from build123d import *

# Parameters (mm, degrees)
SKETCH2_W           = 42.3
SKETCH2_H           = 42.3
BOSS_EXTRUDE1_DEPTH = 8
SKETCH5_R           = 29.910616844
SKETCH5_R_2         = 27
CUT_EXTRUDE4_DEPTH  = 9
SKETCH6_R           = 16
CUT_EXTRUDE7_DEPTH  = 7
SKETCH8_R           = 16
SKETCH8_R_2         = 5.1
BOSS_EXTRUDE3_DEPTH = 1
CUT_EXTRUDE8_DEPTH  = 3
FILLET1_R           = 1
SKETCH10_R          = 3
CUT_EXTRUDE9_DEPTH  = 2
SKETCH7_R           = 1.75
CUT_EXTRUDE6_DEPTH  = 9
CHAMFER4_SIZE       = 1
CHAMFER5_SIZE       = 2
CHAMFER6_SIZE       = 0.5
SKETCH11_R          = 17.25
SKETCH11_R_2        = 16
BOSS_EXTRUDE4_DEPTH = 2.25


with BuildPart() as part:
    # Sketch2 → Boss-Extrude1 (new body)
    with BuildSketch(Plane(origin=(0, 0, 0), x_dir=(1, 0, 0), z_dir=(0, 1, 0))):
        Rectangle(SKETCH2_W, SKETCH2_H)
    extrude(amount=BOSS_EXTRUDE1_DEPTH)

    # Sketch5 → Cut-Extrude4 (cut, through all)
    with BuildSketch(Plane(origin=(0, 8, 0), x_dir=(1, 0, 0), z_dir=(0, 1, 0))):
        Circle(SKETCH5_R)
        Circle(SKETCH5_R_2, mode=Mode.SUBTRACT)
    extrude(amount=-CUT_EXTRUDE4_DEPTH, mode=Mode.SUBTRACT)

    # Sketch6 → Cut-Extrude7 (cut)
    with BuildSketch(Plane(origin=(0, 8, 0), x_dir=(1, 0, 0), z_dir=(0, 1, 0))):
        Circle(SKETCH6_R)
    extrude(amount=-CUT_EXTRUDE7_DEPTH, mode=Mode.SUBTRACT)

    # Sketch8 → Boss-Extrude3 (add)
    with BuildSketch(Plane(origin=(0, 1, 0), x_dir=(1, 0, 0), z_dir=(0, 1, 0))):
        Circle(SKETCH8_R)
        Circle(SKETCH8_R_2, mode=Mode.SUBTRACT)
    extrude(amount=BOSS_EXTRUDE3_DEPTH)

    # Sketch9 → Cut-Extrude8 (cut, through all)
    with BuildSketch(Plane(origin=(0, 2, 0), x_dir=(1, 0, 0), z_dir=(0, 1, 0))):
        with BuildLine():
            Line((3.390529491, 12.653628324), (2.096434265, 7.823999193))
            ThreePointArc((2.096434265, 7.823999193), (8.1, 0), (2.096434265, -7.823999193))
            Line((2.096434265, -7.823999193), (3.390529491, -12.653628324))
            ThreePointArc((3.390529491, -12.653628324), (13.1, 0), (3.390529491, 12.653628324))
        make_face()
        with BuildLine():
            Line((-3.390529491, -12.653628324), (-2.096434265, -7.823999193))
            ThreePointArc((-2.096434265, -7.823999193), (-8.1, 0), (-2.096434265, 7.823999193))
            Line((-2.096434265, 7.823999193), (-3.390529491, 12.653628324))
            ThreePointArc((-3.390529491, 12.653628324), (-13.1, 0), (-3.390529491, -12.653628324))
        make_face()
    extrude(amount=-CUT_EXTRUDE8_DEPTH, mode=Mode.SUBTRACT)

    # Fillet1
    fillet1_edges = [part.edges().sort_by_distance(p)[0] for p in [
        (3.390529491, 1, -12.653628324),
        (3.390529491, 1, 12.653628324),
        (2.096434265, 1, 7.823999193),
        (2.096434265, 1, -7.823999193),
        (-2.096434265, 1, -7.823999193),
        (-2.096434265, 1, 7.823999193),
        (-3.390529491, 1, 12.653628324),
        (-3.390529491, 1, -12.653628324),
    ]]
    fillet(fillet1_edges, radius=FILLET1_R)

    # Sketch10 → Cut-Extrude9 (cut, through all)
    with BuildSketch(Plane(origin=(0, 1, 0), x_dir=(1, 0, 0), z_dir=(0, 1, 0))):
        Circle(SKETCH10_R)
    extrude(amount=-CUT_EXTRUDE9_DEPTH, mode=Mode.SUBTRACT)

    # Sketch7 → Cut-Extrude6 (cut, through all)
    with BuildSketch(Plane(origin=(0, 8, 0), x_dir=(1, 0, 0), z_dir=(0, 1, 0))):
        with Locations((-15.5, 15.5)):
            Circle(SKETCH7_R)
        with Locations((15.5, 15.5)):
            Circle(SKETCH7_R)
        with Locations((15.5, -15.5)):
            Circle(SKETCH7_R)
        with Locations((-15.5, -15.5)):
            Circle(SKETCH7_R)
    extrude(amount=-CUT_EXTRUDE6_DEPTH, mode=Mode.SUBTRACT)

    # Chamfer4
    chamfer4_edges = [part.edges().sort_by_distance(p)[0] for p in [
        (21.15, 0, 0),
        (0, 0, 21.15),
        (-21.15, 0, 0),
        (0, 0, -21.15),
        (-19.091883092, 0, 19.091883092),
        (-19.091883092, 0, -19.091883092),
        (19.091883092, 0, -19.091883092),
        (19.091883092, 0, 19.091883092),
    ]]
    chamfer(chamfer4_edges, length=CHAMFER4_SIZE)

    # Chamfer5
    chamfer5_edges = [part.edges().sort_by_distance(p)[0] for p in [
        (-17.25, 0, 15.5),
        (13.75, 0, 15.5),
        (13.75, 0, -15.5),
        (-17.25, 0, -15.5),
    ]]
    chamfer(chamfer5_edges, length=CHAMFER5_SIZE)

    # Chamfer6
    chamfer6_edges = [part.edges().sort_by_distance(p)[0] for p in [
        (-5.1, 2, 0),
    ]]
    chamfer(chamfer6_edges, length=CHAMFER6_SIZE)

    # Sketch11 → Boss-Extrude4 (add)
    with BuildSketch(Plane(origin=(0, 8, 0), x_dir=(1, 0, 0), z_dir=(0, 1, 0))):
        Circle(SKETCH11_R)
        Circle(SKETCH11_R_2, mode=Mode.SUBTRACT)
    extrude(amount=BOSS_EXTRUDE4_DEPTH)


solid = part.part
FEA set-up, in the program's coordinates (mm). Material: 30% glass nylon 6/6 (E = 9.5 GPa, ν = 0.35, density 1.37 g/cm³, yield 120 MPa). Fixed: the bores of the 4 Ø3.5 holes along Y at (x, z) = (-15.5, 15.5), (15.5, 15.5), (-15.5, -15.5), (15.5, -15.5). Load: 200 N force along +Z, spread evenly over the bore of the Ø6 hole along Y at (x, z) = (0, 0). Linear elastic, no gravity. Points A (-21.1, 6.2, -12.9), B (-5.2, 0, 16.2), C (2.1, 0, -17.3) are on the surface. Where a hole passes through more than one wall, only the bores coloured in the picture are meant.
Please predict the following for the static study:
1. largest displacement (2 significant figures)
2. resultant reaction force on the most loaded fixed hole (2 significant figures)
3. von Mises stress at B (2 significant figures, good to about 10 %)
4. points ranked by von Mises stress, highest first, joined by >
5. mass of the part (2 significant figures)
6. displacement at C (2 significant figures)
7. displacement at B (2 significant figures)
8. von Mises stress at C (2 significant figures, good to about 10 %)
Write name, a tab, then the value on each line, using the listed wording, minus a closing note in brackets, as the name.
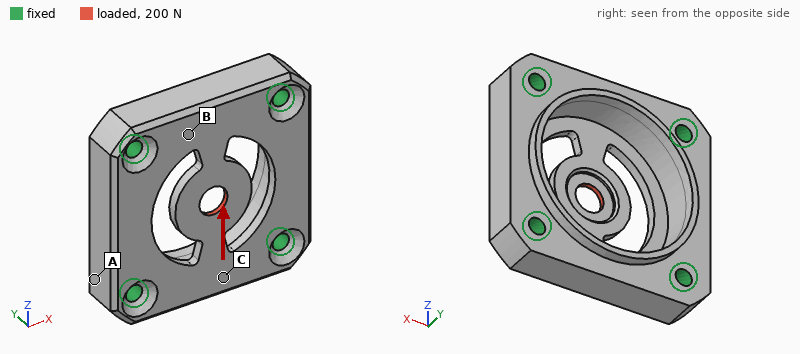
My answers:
largest displacement	25 µm
resultant reaction force on the most loaded fixed hole	52 N
von Mises stress at B	5.1 MPa
points ranked by von Mises stress, highest first, joined by >	B > C > A
mass of the part	11 g
displacement at C	8.9 µm
displacement at B	6.8 µm
von Mises stress at C	3.7 MPa
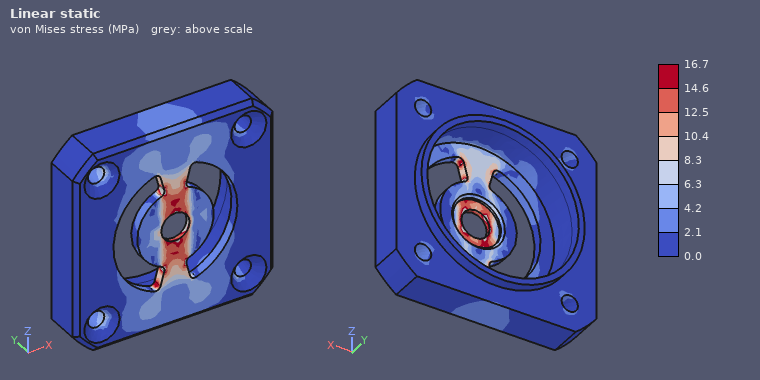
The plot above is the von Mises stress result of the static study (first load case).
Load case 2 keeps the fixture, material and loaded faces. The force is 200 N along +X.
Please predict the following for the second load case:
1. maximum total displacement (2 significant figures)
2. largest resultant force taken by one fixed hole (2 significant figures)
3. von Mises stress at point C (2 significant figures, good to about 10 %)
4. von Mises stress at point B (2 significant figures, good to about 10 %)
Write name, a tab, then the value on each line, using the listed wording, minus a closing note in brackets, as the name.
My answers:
maximum total displacement	0.10 mm
largest resultant force taken by one fixed hole	60 N
von Mises stress at point C	4.0 MPa
von Mises stress at point B	3.7 MPa
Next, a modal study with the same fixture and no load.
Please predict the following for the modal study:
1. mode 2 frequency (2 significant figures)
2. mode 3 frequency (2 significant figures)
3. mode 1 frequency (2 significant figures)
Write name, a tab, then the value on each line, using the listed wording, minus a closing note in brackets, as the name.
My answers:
mode 2 frequency	5300 Hz
mode 3 frequency	11 kHz
mode 1 frequency	4400 Hz
